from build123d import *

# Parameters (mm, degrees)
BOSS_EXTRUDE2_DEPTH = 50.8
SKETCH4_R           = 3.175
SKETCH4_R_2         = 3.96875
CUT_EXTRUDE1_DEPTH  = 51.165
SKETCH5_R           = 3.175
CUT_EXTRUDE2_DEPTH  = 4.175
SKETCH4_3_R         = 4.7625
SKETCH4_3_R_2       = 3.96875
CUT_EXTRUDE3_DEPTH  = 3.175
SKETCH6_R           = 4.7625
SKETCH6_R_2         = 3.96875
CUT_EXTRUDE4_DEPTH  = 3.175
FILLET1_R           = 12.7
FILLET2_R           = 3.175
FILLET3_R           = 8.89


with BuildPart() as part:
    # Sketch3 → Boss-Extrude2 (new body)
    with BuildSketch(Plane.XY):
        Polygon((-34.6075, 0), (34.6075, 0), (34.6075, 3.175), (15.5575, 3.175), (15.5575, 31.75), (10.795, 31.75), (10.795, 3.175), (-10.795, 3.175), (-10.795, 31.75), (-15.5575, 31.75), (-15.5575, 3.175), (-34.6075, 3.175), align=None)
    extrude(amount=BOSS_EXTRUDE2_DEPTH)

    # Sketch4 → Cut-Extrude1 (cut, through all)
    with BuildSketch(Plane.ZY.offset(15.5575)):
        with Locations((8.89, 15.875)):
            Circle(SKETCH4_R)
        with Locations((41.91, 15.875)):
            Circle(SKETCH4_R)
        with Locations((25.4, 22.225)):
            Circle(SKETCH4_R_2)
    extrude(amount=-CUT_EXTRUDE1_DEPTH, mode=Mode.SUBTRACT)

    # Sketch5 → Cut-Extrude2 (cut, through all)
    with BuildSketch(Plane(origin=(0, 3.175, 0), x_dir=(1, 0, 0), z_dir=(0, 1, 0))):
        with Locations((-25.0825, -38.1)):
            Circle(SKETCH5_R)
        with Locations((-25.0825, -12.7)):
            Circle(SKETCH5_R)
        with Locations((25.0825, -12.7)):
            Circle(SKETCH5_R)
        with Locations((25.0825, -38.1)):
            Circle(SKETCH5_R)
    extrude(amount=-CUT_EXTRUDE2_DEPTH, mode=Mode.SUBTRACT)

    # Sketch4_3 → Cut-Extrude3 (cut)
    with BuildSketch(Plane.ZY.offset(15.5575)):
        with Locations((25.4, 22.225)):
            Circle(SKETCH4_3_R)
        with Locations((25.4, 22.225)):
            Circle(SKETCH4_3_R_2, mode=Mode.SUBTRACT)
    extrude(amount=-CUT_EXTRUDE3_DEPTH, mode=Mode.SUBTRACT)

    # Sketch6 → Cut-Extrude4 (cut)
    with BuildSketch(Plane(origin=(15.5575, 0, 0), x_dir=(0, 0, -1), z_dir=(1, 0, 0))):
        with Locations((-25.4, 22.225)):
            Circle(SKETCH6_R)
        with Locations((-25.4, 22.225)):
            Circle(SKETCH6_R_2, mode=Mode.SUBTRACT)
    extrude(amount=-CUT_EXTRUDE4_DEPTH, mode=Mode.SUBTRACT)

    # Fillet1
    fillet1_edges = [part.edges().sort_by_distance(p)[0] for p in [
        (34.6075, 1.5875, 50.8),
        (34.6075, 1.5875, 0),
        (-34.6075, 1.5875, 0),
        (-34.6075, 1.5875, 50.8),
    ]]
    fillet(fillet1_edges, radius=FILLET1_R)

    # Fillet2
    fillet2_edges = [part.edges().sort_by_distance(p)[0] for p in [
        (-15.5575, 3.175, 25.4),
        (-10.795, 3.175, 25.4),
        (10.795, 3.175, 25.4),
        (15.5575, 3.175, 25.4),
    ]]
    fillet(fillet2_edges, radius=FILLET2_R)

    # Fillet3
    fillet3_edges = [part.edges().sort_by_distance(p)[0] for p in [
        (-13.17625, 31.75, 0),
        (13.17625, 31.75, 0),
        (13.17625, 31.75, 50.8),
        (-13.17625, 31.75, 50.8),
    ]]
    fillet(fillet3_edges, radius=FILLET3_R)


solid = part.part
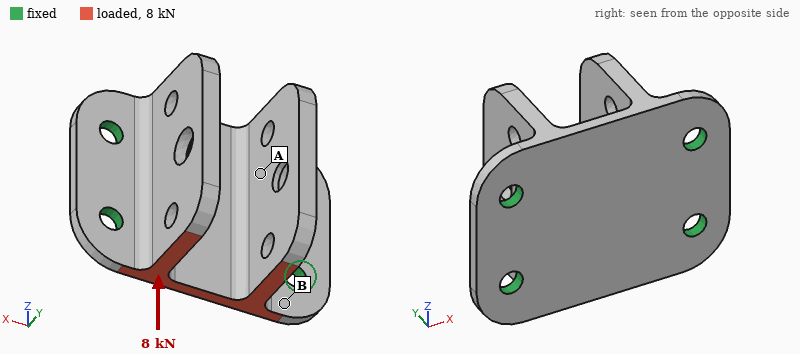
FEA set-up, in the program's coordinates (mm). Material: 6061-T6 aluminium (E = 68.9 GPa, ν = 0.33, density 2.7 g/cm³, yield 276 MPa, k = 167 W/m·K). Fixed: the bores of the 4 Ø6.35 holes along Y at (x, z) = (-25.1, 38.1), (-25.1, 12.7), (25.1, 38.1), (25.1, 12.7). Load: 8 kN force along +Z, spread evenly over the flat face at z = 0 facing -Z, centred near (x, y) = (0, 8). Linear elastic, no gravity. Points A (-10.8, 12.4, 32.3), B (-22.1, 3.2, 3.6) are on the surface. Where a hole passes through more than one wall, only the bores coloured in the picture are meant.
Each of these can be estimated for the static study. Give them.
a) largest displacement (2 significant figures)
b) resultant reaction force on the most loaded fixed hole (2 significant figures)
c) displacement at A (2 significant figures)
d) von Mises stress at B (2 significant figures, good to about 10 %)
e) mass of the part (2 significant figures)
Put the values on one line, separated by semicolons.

93 µm; 2.5 kN; 33 µm; 51 MPa; 62 g
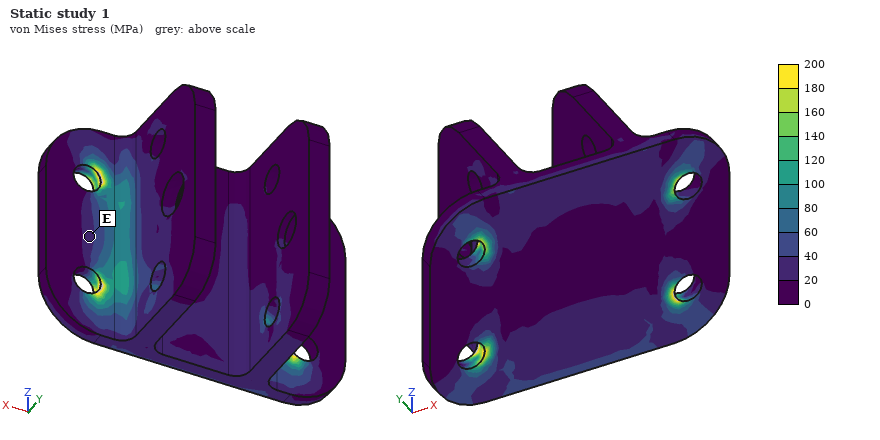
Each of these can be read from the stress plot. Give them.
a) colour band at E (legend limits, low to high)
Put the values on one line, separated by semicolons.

20 to 40 MPa
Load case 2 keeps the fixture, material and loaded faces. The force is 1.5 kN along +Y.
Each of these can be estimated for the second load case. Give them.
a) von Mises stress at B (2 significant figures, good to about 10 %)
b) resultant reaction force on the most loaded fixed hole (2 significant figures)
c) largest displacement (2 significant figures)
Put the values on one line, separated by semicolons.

47 MPa; 1.0 kN; 0.13 mm
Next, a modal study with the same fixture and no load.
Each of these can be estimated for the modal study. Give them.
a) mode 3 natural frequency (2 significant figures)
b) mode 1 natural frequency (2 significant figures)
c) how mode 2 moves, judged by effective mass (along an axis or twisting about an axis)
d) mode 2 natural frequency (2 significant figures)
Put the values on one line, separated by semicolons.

4600 Hz; 2600 Hz; along X; 4200 Hz
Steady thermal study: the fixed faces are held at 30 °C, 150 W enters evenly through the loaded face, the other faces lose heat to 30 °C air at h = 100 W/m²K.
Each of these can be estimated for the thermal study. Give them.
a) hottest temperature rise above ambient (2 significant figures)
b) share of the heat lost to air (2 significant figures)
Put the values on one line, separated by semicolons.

67 K; 19 %
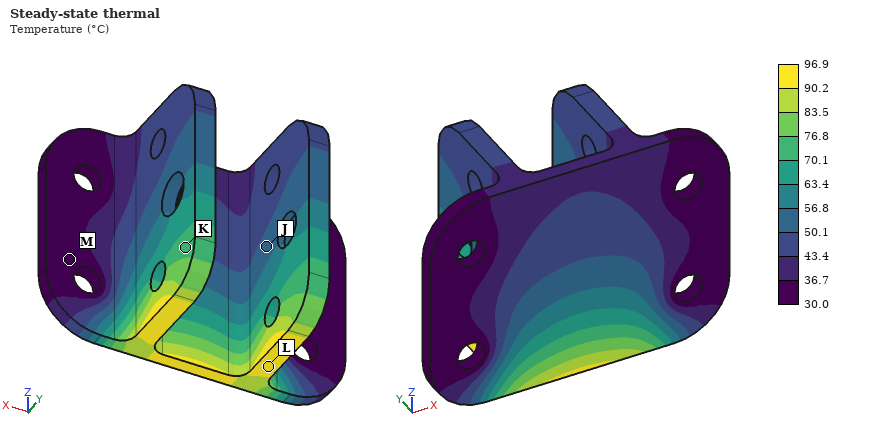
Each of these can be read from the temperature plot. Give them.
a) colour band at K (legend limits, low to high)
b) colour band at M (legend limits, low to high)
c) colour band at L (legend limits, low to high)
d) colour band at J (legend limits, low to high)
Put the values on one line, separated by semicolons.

70.1 to 76.8 °C; 30.0 to 36.7 °C; 90.2 to 96.9 °C; 50.1 to 56.8 °C
